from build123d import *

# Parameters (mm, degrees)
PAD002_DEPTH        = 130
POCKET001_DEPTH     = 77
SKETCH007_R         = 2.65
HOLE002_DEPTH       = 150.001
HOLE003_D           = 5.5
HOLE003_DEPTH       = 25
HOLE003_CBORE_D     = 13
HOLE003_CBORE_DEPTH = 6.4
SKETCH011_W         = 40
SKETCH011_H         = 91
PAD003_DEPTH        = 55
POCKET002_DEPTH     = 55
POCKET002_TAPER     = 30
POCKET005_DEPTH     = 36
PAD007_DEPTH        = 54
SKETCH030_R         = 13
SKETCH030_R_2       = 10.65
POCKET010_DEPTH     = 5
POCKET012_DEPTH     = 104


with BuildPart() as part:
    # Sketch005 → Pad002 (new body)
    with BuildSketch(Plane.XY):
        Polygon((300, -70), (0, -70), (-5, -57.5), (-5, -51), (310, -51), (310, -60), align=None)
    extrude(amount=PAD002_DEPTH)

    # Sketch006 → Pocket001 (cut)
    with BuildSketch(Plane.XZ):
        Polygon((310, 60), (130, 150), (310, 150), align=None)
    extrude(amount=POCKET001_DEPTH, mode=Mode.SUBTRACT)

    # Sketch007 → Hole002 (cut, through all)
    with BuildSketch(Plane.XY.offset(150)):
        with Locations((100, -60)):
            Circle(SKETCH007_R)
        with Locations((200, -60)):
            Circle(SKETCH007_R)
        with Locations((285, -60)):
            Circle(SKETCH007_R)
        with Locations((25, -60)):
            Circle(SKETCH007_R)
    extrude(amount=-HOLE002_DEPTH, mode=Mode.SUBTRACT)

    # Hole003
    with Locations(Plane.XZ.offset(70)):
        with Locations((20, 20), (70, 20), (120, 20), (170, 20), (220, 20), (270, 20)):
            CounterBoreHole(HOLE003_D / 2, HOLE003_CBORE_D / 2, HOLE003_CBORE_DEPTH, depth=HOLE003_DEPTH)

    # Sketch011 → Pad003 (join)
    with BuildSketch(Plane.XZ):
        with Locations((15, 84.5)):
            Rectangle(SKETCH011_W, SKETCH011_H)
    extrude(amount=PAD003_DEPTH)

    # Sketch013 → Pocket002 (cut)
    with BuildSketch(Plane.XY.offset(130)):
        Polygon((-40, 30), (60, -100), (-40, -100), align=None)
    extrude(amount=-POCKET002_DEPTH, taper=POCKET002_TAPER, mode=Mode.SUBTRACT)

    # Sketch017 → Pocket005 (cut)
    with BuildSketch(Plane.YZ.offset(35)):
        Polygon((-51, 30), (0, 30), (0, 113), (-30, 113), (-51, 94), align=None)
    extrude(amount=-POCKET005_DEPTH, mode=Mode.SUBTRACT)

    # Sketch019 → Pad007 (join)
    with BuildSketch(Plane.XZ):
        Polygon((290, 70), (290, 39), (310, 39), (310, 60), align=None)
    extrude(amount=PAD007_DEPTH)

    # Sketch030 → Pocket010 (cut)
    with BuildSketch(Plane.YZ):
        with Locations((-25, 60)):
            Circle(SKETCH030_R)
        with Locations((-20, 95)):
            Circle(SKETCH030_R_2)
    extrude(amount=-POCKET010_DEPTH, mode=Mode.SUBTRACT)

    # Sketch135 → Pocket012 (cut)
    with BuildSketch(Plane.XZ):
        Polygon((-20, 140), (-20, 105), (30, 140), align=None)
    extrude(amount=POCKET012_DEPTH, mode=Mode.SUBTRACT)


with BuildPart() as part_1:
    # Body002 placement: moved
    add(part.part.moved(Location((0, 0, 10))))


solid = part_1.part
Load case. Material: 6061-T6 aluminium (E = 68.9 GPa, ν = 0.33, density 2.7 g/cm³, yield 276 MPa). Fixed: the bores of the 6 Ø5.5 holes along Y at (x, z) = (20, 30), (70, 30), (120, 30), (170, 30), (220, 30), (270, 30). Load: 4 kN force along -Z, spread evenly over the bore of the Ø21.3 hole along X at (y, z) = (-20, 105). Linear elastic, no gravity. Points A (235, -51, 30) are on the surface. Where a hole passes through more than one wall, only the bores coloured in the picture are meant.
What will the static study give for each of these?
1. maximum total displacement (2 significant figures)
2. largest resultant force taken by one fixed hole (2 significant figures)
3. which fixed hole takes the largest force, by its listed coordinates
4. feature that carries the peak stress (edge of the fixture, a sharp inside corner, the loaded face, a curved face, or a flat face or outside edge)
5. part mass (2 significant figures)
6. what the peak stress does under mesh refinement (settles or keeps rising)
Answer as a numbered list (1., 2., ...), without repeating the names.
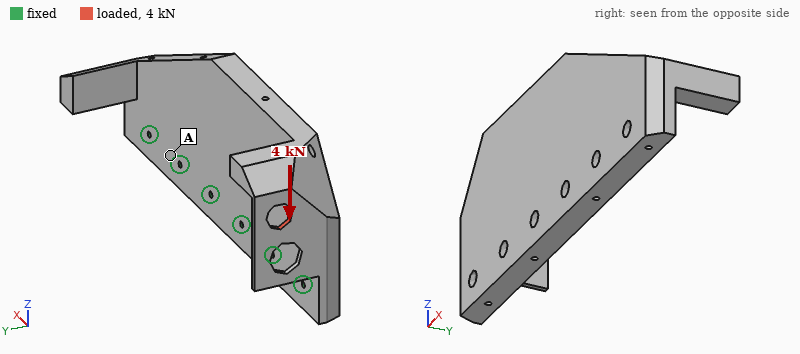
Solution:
1. 0.33 mm
2. 3.7 kN
3. (20, 30)
4. edge of the fixture
5. 1.9 kg
6. keeps rising
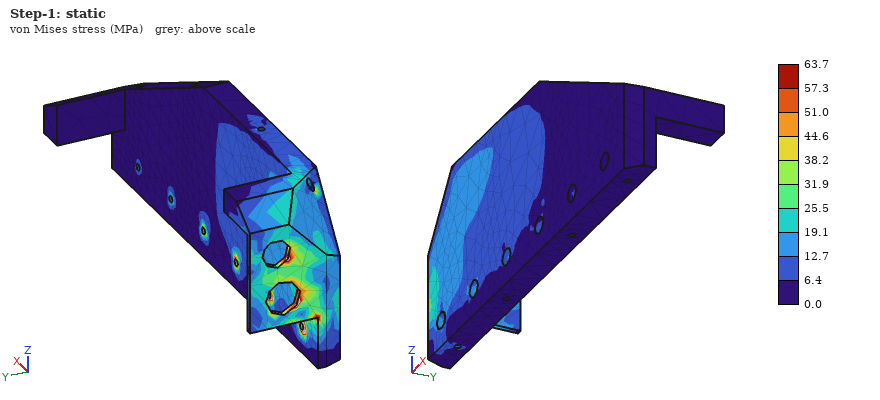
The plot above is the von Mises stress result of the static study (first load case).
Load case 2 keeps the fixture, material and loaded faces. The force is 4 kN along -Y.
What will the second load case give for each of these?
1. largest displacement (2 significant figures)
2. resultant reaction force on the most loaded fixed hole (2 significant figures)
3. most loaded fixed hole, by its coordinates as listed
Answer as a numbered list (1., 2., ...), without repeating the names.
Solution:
1. 0.53 mm
2. 4.2 kN
3. (20, 30)
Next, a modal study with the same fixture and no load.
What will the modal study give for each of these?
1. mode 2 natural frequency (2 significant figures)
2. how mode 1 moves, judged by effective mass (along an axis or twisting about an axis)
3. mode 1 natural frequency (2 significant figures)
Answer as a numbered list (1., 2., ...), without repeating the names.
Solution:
1. 1500 Hz
2. along Y
3. 850 Hz
